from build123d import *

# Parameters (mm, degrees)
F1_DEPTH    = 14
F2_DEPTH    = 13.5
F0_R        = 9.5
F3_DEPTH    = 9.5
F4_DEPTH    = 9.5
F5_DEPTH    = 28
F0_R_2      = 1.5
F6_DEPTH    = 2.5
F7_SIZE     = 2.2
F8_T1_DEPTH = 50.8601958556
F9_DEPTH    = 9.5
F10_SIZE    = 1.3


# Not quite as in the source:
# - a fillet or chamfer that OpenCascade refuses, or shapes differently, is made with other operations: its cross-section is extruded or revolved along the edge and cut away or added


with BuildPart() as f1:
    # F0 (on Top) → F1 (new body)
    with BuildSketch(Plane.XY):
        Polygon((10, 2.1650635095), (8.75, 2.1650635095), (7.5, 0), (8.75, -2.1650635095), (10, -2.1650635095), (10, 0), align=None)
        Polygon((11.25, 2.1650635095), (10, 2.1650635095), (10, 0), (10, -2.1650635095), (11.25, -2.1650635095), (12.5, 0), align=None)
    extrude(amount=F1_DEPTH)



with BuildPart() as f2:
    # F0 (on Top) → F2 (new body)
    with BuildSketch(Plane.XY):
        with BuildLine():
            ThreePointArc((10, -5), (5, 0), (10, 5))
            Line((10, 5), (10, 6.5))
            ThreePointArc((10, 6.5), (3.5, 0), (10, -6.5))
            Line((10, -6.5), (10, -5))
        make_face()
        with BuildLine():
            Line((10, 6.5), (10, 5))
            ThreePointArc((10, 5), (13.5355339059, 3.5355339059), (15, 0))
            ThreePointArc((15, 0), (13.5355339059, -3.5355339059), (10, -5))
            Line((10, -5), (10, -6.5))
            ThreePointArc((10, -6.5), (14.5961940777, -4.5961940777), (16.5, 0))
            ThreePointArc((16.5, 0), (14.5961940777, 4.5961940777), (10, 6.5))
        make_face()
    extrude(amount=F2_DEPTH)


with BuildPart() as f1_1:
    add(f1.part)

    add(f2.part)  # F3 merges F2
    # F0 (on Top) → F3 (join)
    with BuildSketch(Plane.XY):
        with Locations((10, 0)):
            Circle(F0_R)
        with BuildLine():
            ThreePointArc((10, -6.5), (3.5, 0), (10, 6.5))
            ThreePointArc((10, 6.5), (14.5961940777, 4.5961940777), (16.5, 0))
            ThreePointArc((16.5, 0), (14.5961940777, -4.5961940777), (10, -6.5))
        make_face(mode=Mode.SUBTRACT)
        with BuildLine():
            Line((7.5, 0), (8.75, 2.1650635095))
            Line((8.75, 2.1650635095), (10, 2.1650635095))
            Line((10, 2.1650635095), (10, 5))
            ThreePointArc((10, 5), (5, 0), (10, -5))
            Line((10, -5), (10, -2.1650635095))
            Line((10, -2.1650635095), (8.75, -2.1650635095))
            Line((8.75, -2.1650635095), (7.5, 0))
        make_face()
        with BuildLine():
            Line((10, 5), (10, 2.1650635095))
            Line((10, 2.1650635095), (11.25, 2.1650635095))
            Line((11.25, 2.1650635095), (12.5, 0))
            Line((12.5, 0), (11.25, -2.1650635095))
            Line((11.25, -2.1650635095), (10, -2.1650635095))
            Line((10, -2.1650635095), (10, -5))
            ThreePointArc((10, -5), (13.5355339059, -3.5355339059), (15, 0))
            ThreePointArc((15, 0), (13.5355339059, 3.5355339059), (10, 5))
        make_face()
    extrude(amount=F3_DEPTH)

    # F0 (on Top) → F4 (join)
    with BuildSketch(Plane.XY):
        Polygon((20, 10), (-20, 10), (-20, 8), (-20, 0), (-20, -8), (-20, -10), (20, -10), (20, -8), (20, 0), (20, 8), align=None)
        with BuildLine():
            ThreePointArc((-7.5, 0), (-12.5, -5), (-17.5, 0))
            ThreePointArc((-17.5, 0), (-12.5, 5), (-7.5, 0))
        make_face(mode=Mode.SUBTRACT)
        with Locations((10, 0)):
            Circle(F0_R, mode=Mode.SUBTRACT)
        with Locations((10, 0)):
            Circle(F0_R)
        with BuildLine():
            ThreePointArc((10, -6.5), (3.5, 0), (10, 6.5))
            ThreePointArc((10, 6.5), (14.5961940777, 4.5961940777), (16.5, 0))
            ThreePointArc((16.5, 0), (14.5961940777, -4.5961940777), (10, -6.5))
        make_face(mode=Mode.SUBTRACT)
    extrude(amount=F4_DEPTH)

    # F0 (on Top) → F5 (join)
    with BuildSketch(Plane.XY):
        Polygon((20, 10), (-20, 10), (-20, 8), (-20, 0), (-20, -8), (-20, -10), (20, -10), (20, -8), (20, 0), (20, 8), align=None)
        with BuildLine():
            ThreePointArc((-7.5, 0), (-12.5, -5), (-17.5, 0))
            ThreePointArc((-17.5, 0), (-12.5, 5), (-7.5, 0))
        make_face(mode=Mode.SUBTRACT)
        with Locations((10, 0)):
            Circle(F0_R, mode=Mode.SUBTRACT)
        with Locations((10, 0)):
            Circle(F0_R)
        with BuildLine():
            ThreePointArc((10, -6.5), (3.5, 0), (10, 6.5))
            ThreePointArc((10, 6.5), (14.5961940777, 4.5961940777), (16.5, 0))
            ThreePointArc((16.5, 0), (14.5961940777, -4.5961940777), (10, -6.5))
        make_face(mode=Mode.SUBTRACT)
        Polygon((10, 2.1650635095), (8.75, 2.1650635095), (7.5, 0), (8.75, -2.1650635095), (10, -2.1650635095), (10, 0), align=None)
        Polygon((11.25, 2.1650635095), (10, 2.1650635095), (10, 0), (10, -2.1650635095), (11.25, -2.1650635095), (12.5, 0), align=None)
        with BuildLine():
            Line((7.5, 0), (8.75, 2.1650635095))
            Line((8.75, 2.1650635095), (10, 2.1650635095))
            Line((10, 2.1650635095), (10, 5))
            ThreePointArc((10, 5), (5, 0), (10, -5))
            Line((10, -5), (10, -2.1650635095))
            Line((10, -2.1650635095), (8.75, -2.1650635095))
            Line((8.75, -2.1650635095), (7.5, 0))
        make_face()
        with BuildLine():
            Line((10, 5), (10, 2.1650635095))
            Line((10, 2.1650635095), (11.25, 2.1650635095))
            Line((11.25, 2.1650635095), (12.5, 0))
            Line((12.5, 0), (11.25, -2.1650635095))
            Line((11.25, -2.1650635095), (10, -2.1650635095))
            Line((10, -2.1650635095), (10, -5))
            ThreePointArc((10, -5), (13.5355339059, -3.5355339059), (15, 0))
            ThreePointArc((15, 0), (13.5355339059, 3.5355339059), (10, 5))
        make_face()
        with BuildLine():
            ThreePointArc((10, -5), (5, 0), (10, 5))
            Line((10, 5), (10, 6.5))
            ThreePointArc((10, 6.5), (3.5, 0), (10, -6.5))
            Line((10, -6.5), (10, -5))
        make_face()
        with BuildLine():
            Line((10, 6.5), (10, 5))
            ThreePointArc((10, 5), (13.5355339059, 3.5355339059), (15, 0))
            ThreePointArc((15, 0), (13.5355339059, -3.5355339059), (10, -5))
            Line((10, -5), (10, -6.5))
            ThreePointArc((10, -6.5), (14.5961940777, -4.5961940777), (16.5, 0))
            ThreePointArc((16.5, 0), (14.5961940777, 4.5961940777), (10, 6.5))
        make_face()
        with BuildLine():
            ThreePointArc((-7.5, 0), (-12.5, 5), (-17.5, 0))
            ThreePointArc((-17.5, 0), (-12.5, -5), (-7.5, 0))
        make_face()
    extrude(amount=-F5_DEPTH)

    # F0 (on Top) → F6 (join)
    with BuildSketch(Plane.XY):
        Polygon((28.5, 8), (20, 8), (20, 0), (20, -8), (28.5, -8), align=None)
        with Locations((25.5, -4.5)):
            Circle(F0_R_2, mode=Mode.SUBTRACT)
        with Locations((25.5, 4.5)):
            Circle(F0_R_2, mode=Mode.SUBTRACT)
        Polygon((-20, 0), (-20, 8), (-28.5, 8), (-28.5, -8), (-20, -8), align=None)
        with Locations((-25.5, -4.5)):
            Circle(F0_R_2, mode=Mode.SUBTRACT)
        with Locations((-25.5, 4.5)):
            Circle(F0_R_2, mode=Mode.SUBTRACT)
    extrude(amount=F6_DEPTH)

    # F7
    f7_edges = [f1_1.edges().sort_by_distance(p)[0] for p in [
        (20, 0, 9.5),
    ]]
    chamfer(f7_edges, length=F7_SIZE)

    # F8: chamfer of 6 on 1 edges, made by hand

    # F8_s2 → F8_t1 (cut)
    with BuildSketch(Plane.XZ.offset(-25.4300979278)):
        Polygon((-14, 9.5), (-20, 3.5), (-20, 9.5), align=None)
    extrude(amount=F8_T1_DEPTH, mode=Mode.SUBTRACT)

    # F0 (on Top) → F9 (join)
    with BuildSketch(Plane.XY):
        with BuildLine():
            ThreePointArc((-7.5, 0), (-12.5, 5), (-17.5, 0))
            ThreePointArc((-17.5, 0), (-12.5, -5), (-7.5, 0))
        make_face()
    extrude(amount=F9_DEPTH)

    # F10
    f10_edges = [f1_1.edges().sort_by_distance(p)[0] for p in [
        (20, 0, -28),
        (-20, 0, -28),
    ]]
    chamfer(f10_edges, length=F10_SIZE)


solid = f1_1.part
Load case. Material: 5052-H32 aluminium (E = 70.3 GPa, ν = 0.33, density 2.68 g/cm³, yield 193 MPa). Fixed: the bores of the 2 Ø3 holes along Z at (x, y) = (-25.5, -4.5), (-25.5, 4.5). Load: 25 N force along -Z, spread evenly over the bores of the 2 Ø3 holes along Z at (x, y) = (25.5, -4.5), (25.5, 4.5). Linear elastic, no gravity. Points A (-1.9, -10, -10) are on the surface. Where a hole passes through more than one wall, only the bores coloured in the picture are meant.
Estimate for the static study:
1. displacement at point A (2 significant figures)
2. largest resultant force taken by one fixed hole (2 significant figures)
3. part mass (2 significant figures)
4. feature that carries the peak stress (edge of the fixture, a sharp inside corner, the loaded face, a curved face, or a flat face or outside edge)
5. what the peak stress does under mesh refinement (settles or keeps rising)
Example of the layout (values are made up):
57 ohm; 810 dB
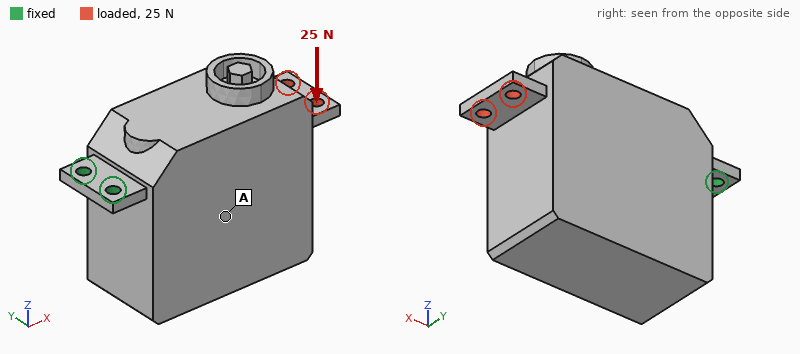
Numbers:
0.097 mm; 13 N; 82 g; edge of the fixture; keeps rising
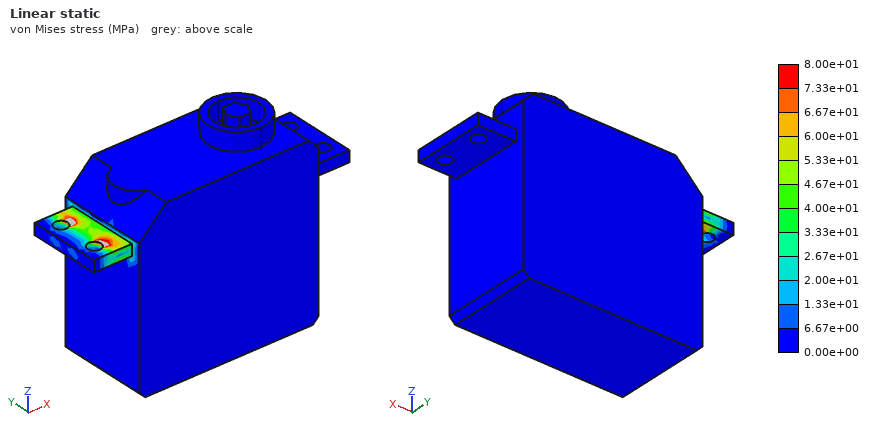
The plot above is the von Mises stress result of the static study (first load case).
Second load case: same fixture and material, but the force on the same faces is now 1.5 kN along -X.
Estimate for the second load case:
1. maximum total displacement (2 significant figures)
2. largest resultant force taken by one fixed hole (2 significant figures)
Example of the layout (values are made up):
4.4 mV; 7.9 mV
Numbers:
14 µm; 750 N
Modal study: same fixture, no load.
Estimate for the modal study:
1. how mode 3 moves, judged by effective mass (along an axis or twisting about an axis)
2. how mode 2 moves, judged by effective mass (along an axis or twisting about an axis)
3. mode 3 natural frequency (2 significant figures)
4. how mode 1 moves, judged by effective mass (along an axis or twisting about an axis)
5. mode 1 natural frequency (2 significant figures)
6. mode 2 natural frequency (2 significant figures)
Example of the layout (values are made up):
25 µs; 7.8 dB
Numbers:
along Y; along Y; 2500 Hz; along Z; 320 Hz; 1300 Hz
